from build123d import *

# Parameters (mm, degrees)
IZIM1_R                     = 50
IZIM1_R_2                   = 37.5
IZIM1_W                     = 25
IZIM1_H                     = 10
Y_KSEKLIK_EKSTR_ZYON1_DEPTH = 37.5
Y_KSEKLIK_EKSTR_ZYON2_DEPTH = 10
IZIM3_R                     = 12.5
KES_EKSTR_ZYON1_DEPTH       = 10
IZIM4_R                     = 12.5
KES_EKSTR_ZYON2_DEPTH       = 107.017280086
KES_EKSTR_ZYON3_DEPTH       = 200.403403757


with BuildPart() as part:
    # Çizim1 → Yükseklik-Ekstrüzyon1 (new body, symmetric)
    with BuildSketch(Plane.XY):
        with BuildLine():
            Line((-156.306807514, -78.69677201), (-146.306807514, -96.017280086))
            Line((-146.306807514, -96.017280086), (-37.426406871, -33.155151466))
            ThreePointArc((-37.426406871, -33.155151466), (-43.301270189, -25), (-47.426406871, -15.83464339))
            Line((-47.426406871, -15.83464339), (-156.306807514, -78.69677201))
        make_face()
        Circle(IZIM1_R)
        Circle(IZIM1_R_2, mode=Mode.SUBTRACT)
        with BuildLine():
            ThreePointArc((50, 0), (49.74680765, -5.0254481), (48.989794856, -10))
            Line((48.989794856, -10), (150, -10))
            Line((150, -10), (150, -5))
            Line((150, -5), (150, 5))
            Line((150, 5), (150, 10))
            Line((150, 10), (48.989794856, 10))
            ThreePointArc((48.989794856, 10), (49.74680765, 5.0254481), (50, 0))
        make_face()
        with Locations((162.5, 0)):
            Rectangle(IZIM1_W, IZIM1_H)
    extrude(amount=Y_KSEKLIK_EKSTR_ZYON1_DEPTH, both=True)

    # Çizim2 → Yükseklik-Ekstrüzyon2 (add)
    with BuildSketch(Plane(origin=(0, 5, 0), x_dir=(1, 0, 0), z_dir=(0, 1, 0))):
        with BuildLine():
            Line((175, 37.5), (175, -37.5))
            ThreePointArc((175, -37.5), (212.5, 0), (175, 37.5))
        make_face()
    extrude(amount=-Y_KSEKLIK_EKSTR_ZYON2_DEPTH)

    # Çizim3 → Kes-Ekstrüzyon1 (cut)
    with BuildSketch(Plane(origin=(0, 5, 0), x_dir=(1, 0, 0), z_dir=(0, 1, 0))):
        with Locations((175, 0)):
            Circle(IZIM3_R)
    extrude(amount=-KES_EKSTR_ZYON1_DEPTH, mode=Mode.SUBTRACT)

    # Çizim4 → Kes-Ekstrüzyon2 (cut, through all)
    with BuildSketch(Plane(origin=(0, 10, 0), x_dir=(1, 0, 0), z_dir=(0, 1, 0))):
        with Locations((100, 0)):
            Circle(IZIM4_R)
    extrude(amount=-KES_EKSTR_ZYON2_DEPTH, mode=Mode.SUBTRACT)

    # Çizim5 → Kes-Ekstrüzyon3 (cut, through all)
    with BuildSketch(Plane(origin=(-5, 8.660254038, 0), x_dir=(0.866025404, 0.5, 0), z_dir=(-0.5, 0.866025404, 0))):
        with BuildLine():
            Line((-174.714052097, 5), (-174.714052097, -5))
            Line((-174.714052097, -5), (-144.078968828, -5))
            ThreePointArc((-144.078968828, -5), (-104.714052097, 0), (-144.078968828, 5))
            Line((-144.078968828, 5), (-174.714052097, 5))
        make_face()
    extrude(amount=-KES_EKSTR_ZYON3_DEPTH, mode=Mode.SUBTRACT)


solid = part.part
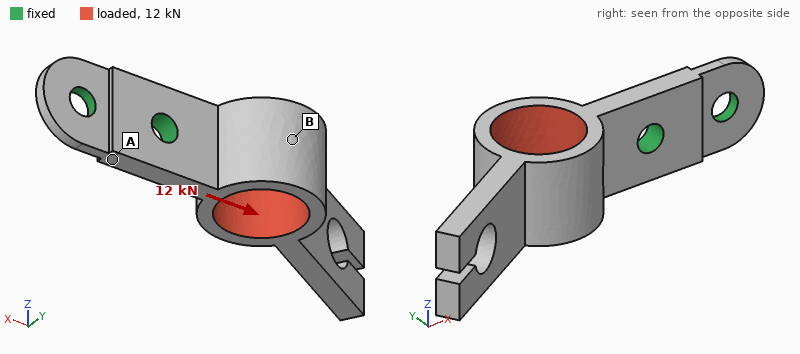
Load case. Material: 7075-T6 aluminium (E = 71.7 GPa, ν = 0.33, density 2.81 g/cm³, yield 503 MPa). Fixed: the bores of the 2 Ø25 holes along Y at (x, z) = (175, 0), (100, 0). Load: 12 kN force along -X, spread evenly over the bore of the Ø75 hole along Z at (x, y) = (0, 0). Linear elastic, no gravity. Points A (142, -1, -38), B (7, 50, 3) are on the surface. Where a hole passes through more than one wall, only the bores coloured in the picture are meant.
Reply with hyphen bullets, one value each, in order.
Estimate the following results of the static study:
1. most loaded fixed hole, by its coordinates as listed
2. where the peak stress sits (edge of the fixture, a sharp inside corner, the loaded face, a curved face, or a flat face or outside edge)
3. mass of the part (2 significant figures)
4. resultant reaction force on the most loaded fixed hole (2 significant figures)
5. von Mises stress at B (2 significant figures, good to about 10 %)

- (100, 0)
- the loaded face
- 1.7 kg
- 11 kN
- 17 MPa
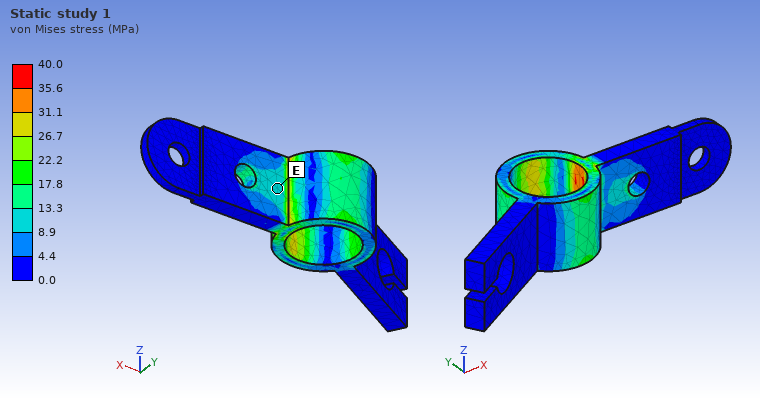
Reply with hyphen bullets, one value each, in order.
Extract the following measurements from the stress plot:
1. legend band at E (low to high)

- 8.9 to 13.3 MPa
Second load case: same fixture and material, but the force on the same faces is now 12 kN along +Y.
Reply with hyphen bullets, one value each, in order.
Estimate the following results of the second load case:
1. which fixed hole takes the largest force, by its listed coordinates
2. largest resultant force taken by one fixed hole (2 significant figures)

- (100, 0)
- 13 kN
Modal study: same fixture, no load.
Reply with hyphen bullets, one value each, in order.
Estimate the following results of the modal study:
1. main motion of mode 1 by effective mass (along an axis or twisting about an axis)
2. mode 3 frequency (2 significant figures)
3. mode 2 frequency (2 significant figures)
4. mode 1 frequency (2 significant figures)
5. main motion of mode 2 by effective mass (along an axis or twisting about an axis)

- along Y
- 1200 Hz
- 480 Hz
- 260 Hz
- along Z
